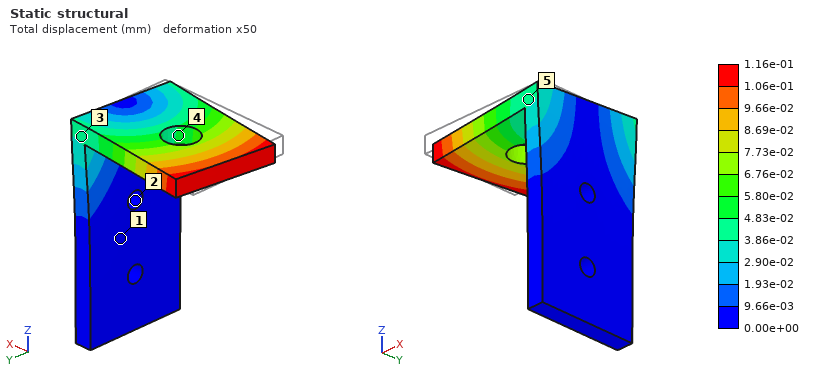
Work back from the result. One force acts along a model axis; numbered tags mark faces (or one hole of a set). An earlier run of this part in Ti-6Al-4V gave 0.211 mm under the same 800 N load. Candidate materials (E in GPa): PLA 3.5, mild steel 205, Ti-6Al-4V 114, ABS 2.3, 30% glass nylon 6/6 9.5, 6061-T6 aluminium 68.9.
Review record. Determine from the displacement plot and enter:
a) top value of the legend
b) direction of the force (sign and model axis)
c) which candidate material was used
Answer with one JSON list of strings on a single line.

["1.16e-01 mm", "+Y", "mild steel"]
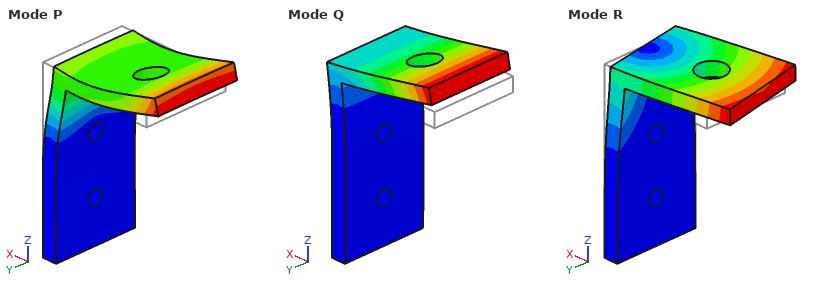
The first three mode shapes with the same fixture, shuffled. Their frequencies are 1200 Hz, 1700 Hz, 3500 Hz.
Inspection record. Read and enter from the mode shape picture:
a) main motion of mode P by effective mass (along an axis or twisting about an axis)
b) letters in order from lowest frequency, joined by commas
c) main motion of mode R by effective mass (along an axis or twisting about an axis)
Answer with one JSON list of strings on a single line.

["along X", "Q, R, P", "along Y"]
